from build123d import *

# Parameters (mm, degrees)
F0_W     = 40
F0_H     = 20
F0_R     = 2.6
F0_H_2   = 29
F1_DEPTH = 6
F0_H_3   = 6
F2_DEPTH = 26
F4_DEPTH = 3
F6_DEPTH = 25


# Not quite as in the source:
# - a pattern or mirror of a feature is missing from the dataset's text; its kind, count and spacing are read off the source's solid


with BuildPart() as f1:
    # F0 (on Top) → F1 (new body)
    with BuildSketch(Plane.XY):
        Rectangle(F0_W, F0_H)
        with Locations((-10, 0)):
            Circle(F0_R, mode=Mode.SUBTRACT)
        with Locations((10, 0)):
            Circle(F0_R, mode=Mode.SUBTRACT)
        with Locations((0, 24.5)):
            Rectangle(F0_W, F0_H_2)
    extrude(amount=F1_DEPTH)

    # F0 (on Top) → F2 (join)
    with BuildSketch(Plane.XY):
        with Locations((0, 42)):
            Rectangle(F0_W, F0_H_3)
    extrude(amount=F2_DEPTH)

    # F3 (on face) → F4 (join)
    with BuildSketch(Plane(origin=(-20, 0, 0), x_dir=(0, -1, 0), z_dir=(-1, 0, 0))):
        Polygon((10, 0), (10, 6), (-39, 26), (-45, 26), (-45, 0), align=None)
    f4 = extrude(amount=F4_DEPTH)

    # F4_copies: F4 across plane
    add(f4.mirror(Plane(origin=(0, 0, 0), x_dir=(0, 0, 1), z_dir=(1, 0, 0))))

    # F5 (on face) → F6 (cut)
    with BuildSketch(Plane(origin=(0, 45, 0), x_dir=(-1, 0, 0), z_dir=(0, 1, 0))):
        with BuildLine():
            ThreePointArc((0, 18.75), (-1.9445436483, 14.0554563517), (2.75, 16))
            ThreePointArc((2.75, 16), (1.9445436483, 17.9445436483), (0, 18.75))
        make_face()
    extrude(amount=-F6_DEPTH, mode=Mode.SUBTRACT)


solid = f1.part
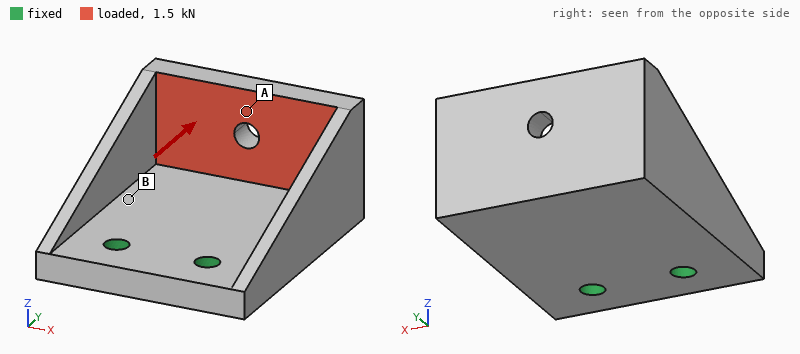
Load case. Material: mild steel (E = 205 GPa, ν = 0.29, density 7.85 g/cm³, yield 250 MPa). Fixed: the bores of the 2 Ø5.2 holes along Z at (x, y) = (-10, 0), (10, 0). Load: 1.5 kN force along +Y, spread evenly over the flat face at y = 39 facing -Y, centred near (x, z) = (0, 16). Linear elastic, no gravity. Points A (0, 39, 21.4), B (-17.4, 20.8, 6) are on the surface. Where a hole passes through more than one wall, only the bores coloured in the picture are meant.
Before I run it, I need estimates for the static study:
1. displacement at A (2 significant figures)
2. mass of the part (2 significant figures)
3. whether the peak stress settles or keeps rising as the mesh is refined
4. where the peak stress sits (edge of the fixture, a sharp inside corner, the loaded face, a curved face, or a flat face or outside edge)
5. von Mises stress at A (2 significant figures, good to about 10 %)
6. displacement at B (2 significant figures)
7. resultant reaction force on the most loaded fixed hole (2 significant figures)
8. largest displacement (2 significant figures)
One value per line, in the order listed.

51 µm
180 g
keeps rising
edge of the fixture
26 MPa
16 µm
750 N
64 µm
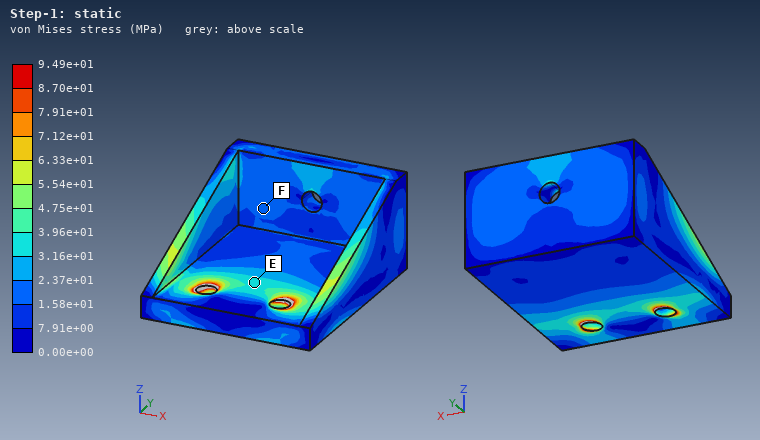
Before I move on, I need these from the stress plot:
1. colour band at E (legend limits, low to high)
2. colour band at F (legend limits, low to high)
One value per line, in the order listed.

3.16e+01 to 3.96e+01 MPa
1.58e+01 to 2.37e+01 MPa
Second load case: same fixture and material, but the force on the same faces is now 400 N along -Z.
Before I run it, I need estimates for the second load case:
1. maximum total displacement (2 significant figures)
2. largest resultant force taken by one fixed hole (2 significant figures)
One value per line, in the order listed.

38 µm
200 N
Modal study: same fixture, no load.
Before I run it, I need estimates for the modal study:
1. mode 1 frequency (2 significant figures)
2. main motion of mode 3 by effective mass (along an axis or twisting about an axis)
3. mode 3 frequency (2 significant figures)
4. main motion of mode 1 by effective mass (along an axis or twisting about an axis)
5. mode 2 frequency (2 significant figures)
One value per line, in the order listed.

1800 Hz
along X
6600 Hz
along Z
3100 Hz
